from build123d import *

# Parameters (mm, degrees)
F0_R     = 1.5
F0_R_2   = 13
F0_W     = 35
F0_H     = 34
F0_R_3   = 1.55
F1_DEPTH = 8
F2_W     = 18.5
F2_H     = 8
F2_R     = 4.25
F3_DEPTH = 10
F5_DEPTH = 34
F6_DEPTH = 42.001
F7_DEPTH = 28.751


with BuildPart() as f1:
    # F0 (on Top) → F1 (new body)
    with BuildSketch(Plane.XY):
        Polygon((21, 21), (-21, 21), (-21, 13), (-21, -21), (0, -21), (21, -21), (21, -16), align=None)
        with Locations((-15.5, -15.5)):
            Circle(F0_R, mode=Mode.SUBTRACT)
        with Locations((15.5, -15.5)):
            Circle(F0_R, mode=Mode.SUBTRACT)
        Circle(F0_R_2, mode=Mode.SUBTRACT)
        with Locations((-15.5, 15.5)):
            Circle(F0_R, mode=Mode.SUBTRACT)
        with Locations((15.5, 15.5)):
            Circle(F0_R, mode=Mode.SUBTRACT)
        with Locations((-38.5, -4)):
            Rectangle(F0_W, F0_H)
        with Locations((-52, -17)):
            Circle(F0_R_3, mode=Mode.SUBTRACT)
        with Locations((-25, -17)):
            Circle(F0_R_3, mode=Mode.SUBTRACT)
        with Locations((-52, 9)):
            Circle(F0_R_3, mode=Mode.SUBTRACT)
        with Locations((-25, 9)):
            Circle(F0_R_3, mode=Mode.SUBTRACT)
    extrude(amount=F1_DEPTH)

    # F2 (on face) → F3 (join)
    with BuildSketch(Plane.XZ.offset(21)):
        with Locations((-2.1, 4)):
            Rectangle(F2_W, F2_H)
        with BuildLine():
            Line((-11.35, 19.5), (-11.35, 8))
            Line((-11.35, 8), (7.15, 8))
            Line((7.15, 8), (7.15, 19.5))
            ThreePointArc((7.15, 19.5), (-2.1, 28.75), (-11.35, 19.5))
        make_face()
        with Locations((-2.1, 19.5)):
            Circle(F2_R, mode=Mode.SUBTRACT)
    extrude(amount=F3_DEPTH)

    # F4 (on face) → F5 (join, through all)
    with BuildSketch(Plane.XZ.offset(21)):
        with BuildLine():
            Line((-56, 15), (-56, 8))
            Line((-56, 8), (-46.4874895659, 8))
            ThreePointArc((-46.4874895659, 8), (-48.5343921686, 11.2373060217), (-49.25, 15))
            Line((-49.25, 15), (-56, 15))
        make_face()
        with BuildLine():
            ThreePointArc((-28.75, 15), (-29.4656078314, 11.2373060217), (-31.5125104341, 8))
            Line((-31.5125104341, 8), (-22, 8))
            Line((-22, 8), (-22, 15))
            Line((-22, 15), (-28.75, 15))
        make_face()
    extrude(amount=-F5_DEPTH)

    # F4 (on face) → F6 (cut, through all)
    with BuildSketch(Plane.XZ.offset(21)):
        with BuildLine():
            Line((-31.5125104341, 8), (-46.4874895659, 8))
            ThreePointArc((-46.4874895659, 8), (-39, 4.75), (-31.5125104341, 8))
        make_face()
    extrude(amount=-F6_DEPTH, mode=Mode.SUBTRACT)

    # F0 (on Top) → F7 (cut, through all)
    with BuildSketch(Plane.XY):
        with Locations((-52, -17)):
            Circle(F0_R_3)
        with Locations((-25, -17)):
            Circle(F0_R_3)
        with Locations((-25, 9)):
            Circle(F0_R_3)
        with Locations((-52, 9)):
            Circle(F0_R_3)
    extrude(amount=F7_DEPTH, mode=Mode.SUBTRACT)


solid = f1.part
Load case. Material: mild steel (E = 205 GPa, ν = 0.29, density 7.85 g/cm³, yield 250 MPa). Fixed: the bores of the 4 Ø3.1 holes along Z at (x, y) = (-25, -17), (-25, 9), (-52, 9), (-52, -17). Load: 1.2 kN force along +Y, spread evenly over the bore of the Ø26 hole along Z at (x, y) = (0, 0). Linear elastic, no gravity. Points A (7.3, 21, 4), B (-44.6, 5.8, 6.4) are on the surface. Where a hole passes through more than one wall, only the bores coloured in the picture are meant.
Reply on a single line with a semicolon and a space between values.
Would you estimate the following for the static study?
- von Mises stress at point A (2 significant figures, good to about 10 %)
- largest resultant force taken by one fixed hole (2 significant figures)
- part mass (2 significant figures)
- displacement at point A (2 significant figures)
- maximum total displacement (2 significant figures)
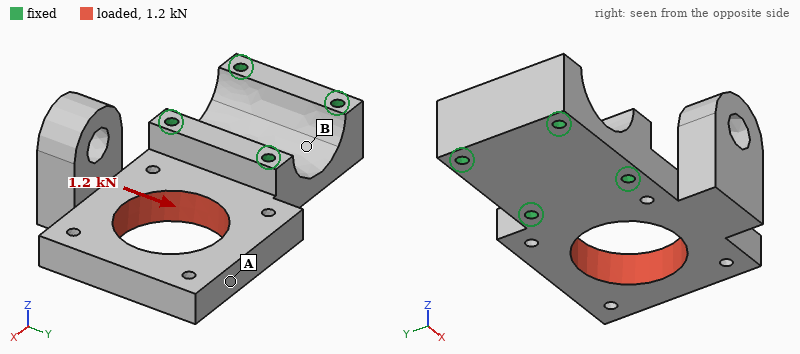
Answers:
14 MPa; 1.2 kN; 200 g; 11 µm; 12 µm
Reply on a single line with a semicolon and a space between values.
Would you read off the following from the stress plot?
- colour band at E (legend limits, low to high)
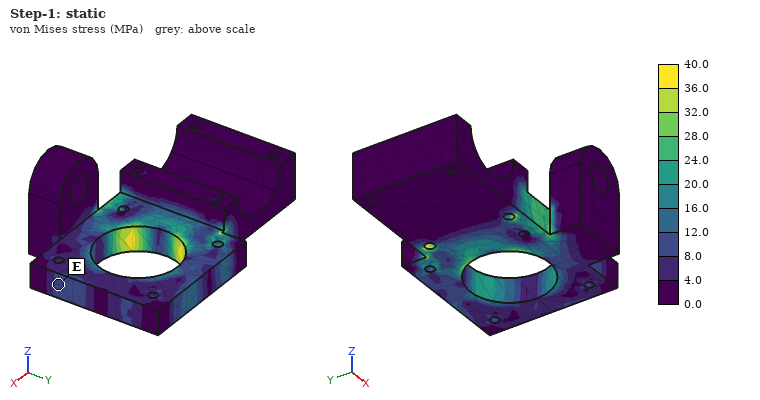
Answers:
8.0 to 12.0 MPa
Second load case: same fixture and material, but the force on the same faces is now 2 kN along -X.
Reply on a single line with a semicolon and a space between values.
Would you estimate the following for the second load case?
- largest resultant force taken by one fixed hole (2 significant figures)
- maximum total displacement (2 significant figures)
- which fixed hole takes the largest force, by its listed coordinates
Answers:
1.2 kN; 5.0 µm; (-25, 9)
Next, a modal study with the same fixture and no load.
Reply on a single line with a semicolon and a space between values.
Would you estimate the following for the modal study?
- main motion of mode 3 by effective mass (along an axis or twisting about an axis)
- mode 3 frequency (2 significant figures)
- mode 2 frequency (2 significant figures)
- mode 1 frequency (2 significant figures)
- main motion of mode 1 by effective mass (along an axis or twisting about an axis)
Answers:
along Y; 5200 Hz; 3700 Hz; 2300 Hz; along Z
